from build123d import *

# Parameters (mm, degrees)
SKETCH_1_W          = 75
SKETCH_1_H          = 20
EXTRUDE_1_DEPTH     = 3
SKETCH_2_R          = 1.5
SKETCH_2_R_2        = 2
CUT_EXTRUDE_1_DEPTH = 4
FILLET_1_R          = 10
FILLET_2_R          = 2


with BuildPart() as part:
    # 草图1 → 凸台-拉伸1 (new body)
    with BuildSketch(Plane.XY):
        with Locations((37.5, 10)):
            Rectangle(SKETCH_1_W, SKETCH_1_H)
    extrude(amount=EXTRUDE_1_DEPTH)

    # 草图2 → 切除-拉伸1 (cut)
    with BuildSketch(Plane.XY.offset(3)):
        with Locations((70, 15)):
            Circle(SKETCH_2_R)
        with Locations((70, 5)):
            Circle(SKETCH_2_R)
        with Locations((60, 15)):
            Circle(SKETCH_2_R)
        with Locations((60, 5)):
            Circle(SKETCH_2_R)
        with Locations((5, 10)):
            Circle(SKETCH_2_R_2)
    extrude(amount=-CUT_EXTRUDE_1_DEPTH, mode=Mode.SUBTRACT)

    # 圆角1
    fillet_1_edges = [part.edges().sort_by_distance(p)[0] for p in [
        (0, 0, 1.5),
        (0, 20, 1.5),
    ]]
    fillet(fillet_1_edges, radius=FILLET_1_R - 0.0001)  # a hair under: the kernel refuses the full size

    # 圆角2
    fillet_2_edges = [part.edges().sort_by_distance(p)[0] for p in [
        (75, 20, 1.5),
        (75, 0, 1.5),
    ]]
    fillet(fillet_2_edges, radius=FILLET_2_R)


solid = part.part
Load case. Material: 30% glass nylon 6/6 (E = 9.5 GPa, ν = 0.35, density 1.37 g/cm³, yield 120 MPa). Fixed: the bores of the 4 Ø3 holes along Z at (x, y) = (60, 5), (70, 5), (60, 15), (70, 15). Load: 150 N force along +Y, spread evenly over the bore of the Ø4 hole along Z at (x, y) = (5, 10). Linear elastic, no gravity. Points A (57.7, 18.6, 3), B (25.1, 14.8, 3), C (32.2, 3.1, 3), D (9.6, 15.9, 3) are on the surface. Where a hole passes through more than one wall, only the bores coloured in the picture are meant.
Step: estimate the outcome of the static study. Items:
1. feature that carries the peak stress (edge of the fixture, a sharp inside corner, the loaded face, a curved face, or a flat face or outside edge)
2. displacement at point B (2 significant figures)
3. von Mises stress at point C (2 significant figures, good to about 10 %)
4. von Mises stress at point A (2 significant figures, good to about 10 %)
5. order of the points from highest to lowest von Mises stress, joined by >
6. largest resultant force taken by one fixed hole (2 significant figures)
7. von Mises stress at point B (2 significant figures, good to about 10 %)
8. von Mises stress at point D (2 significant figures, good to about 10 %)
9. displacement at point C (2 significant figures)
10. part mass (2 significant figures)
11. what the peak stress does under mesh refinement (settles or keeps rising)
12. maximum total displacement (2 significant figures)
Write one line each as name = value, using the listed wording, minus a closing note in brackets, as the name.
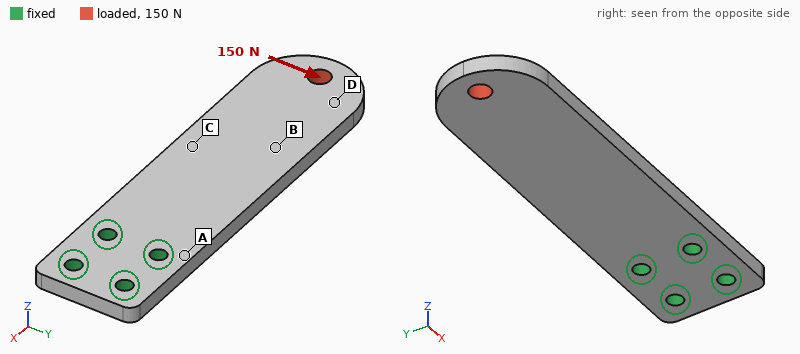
feature that carries the peak stress = edge of the fixture
displacement at point B = 0.26 mm
von Mises stress at point C = 14 MPa
von Mises stress at point A = 26 MPa
order of the points from highest to lowest von Mises stress, joined by > = A > C > B > D
largest resultant force taken by one fixed hole = 570 N
von Mises stress at point B = 8.8 MPa
von Mises stress at point D = 4.4 MPa
displacement at point C = 0.19 mm
part mass = 5.8 g
what the peak stress does under mesh refinement = keeps rising
maximum total displacement = 0.58 mm
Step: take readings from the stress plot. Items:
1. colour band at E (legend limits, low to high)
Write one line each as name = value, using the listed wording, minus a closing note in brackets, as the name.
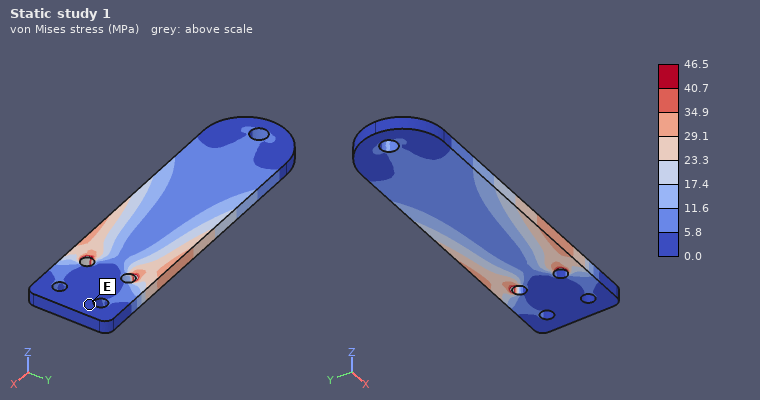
colour band at E = 0.0 to 5.8 MPa
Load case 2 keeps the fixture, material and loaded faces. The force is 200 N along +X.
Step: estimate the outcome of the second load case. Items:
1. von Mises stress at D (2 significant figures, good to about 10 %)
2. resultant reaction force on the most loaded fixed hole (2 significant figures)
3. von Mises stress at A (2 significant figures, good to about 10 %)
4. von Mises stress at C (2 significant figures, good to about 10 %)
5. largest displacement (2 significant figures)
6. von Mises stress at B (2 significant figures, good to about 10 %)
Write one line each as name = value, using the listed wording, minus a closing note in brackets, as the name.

von Mises stress at D = 3.6 MPa
resultant reaction force on the most loaded fixed hole = 89 N
von Mises stress at A = 2.3 MPa
von Mises stress at C = 3.3 MPa
largest displacement = 25 µm
von Mises stress at B = 3.3 MPa
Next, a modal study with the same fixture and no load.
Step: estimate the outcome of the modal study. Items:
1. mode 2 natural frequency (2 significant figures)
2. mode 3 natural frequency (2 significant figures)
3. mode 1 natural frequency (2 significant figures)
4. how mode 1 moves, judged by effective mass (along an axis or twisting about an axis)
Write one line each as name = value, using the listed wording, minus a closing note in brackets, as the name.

mode 2 natural frequency = 2200 Hz
mode 3 natural frequency = 2300 Hz
mode 1 natural frequency = 400 Hz
how mode 1 moves, judged by effective mass = along Z
